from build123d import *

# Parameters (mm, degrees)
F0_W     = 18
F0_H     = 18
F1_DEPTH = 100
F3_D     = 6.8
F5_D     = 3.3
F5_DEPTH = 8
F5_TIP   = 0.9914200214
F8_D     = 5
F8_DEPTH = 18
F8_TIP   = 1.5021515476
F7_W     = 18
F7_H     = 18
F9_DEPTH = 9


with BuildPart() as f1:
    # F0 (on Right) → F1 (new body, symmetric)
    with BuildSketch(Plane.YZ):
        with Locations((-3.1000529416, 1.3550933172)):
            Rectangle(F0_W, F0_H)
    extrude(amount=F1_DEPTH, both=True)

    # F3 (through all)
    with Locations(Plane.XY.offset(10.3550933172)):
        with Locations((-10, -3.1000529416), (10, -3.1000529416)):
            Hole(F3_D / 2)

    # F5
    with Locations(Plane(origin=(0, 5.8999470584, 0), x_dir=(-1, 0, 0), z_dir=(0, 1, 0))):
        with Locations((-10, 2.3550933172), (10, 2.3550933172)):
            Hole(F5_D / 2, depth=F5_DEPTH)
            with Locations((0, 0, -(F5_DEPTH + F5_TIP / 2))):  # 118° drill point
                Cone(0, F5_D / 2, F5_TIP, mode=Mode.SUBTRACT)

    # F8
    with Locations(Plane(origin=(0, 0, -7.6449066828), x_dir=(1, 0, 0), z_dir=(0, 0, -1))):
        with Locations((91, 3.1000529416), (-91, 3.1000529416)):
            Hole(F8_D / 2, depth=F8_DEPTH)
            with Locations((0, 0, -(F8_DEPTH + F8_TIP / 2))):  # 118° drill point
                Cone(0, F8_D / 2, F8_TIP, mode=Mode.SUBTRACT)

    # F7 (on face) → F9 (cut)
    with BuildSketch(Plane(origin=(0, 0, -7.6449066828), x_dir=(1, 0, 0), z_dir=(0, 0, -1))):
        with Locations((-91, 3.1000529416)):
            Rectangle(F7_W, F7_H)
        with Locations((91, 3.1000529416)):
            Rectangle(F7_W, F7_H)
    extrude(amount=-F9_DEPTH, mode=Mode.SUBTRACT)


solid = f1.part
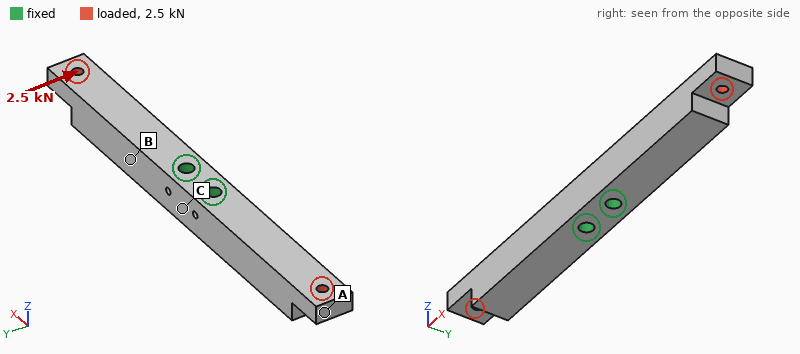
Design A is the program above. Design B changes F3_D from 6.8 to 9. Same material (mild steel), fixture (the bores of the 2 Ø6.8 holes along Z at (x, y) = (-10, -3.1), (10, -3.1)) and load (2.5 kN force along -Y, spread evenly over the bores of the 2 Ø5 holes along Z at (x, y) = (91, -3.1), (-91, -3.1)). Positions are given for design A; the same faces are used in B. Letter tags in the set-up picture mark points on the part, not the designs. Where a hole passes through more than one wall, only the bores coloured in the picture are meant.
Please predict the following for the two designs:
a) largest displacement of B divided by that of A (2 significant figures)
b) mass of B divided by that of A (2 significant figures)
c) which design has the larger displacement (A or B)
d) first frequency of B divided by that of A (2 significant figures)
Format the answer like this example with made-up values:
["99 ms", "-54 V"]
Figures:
["0.92", "0.98", "A", "1.1"]
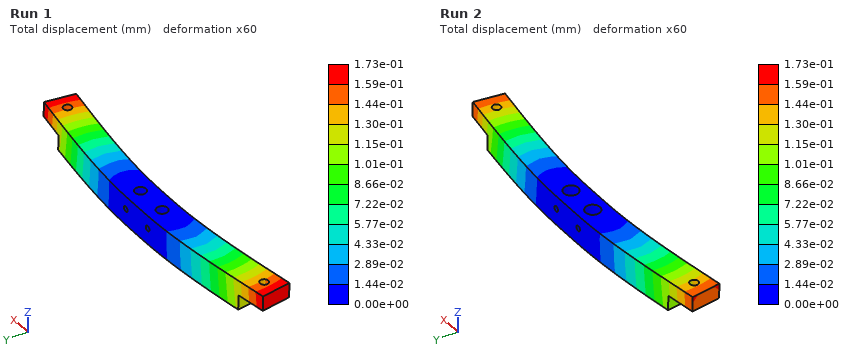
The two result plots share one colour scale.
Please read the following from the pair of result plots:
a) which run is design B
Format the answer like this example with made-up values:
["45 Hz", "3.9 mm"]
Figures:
["Run 2"]
